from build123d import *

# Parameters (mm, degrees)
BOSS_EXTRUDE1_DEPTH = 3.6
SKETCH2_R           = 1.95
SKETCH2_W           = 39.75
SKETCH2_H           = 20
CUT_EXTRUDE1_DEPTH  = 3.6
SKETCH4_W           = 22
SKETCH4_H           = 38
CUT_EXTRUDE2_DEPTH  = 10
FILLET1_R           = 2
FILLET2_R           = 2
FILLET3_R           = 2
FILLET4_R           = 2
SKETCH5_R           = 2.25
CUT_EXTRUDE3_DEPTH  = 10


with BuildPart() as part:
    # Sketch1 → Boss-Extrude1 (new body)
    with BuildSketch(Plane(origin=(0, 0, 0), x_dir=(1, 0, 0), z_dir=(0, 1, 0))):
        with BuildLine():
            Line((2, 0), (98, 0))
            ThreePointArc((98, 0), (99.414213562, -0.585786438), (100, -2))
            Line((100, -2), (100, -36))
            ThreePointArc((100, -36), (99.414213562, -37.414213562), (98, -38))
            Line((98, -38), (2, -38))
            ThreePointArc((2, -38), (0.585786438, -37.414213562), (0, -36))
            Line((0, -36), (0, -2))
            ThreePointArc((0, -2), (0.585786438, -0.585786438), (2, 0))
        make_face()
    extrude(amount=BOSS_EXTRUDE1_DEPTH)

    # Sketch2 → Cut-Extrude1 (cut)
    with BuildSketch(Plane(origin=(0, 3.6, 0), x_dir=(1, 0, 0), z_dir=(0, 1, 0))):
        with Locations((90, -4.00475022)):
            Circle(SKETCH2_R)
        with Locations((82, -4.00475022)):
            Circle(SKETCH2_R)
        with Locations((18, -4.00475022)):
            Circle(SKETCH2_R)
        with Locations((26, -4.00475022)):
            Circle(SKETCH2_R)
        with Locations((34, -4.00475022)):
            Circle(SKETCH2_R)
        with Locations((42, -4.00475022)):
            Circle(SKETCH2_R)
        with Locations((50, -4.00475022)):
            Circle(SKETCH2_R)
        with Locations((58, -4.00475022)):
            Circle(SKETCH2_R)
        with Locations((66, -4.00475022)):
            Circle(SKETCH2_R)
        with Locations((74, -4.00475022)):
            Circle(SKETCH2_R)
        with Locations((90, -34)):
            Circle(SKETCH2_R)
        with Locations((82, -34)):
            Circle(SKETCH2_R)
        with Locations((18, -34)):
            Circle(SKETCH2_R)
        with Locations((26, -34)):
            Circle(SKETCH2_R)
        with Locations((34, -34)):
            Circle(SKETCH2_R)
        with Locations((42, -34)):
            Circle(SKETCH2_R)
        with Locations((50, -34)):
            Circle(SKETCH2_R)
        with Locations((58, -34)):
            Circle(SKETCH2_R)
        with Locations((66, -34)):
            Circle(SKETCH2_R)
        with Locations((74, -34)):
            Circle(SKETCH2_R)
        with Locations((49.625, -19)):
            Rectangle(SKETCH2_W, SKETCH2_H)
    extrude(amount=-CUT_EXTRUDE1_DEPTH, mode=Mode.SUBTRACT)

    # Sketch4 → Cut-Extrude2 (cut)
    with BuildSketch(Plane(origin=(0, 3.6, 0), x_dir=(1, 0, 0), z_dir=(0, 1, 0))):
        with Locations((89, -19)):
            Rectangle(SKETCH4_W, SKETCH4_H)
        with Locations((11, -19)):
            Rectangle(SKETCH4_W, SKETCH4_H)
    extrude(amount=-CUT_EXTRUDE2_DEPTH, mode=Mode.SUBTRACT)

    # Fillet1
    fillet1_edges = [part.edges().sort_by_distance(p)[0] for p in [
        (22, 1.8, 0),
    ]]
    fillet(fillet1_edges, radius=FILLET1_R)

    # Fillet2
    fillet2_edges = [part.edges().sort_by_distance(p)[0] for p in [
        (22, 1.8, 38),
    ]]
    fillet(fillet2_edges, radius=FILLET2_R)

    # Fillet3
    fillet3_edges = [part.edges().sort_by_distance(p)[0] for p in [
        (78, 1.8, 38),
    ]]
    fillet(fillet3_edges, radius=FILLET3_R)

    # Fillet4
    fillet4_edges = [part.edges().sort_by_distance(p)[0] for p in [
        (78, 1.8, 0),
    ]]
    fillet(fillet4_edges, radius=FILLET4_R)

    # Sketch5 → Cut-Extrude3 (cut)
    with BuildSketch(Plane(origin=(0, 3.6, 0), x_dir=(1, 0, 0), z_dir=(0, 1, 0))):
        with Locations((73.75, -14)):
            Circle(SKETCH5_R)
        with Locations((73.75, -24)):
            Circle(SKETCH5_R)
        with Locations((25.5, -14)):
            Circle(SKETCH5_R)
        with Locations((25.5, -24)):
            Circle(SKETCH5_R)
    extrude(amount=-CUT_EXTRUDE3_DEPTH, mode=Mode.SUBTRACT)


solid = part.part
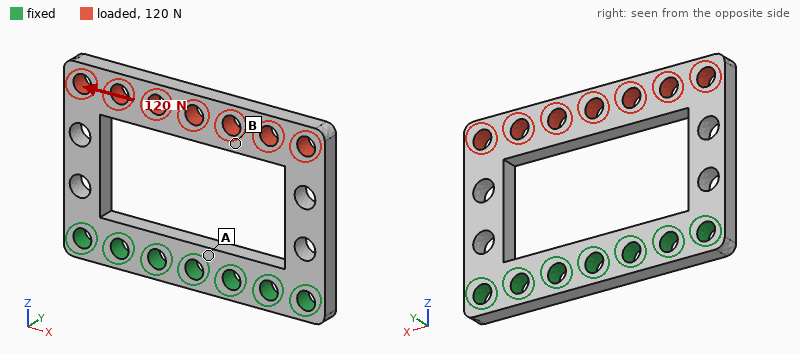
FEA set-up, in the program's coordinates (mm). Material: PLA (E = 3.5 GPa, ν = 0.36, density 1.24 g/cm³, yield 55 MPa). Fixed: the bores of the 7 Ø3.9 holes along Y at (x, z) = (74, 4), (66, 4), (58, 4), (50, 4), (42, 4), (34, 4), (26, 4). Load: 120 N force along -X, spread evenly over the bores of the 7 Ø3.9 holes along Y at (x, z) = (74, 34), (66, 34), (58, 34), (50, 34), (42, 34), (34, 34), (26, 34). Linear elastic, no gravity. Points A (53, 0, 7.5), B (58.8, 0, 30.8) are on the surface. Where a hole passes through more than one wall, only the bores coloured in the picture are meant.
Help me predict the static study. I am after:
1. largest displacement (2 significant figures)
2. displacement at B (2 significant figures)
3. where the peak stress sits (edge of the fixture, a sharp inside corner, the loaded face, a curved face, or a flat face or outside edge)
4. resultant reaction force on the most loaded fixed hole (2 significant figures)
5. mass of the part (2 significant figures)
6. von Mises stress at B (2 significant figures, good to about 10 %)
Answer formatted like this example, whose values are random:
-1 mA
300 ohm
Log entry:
0.46 mm
0.43 mm
a curved face
130 N
4.9 g
6.9 MPa
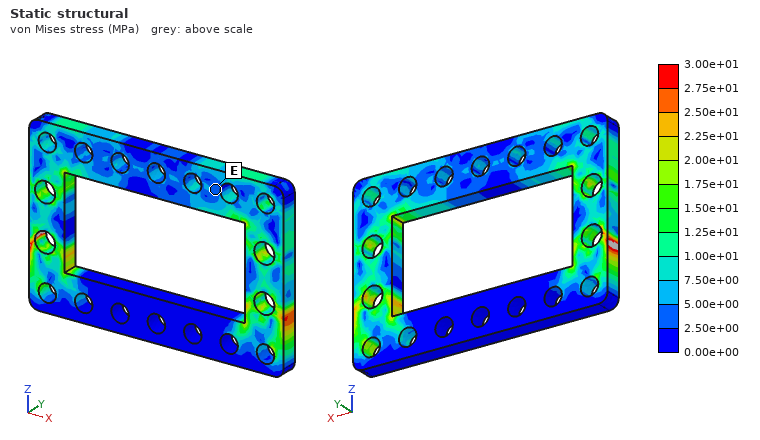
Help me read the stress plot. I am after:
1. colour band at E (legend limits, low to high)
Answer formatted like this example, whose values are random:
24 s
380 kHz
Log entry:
2.50e+00 to 5.00e+00 MPa
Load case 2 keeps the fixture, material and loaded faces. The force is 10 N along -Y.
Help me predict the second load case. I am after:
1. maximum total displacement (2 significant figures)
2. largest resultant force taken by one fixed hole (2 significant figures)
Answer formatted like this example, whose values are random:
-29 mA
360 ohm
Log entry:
0.68 mm
4.4 N
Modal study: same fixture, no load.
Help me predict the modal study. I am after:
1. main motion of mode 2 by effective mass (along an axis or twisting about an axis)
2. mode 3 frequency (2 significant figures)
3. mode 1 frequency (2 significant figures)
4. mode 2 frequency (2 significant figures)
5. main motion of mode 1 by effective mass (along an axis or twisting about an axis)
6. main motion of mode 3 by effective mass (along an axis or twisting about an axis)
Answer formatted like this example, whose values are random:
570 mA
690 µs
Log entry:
twisting about Z
1800 Hz
500 Hz
1000 Hz
along Y
along X
